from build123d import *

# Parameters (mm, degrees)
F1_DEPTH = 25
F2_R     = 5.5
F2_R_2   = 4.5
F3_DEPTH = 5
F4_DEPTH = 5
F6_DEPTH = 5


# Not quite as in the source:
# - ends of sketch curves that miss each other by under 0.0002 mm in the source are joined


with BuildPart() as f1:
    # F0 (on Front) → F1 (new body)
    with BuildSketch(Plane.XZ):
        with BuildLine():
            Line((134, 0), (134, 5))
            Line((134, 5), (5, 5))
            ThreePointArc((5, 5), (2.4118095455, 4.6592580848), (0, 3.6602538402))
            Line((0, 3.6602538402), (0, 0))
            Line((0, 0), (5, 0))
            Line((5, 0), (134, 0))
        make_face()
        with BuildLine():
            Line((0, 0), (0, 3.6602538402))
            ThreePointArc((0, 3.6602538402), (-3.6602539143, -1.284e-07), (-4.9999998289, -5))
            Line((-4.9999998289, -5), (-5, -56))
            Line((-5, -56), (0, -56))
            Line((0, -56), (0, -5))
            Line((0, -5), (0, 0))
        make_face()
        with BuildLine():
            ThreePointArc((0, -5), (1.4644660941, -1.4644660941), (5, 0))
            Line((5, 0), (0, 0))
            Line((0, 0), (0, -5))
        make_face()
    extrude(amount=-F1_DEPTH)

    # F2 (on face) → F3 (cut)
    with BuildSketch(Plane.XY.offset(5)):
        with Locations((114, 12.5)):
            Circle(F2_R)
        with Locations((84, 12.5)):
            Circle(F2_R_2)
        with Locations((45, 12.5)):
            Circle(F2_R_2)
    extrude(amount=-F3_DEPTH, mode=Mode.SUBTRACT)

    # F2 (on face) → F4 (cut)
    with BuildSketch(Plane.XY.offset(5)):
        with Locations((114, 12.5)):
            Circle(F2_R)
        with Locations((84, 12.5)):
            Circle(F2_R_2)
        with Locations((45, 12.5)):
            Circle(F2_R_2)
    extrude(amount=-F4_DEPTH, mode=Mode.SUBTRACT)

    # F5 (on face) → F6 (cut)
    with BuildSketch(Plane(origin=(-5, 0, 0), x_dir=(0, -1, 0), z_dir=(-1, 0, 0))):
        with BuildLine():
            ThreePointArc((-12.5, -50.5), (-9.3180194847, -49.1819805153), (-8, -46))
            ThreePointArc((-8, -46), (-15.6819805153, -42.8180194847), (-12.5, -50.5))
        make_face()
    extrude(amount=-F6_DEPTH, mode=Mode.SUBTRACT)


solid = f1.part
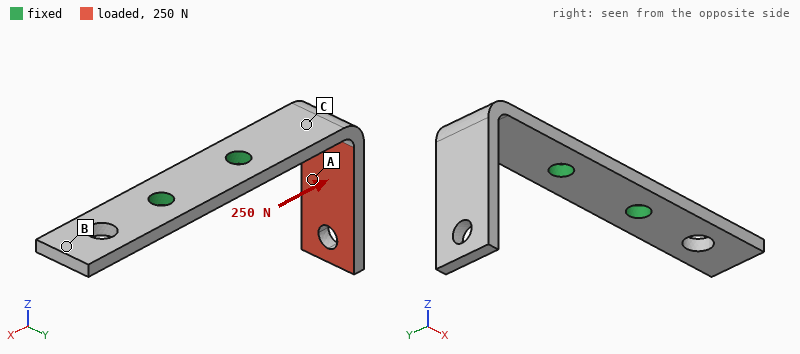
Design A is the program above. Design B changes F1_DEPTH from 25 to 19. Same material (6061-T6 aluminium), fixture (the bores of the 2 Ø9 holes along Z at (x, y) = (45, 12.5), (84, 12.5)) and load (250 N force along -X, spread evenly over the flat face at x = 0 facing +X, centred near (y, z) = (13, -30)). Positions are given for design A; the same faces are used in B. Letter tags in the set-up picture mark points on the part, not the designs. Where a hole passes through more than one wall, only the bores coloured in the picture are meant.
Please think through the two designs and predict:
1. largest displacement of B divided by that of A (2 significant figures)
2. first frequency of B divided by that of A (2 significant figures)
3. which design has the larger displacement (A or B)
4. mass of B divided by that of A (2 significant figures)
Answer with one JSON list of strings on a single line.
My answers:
["1.3", "1.0", "B", "0.74"]
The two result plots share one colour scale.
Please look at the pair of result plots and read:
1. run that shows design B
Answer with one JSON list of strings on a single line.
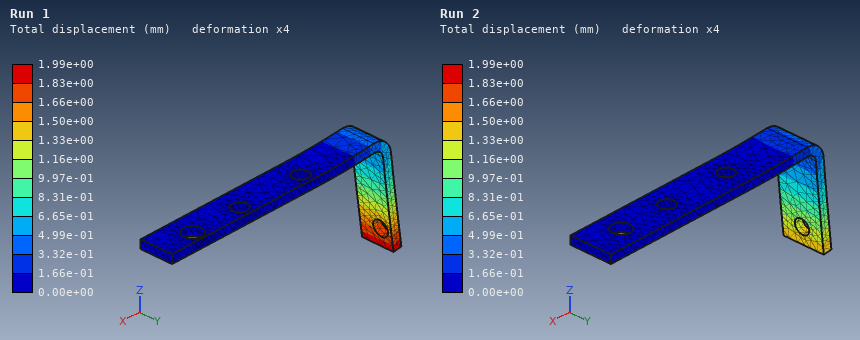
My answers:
["Run 1"]
